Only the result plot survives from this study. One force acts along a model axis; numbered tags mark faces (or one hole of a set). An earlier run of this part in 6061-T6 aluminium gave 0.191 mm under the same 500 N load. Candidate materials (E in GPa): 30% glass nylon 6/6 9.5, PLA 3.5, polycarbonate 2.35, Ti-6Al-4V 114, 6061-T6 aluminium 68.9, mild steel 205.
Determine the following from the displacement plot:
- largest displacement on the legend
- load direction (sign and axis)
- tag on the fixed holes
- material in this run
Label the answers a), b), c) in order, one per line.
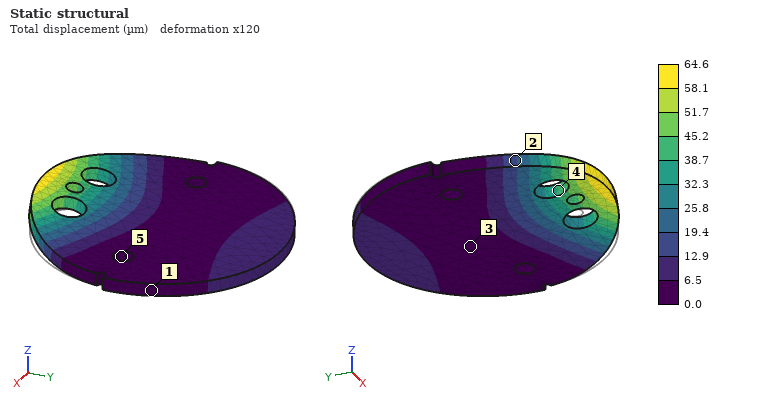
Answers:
a) 64.6 µm
b) +Z
c) 5
d) mild steel
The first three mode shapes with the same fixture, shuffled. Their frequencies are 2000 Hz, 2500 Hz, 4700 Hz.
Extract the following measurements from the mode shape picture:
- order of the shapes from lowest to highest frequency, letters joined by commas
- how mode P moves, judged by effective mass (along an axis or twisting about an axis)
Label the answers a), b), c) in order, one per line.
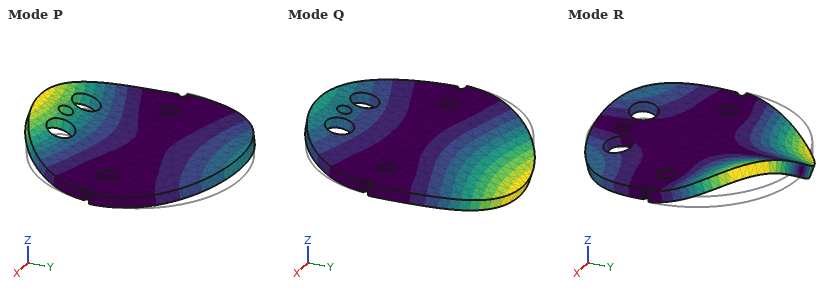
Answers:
a) Q, P, R
b) along Z
